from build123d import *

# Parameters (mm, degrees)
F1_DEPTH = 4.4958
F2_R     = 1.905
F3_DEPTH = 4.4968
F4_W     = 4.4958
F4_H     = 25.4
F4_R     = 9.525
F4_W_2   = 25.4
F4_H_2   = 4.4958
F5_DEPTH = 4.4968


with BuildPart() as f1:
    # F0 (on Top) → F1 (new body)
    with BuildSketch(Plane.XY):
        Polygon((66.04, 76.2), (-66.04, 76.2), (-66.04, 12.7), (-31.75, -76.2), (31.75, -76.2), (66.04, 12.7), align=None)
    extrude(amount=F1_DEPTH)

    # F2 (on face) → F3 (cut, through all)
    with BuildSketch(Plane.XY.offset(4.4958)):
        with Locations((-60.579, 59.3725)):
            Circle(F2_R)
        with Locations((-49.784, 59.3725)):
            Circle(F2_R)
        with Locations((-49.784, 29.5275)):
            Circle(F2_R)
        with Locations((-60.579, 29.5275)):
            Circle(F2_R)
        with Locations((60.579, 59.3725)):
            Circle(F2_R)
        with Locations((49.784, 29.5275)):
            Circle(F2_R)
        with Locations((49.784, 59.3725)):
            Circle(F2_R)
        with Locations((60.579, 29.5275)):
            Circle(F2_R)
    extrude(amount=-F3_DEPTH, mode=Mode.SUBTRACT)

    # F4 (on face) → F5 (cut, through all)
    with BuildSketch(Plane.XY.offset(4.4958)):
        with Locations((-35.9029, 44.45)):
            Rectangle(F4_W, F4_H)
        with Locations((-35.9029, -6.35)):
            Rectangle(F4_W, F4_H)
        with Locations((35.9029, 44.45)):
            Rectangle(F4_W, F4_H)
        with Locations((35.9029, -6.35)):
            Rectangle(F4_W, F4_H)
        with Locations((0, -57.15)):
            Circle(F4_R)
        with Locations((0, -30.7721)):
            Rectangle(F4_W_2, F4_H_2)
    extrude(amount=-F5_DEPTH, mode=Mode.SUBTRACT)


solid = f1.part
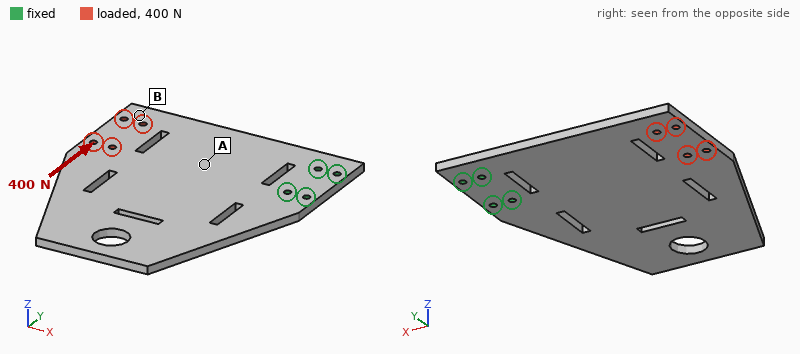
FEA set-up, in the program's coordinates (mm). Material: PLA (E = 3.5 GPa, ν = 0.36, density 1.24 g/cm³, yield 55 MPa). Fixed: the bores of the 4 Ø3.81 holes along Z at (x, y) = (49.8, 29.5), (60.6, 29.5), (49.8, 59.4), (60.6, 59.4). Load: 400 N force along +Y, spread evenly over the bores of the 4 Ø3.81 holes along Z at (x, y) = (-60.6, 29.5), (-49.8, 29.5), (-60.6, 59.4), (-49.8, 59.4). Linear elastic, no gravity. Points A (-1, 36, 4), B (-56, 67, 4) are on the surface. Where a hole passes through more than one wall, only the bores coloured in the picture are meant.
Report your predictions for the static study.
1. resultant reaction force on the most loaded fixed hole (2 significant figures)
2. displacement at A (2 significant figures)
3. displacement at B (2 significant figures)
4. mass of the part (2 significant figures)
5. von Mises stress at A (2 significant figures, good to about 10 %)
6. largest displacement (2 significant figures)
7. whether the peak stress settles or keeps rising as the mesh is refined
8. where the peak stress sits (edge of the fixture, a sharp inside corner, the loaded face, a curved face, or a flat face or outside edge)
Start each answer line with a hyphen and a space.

- 910 N
- 0.38 mm
- 0.84 mm
- 90 g
- 3.7 MPa
- 1.0 mm
- keeps rising
- edge of the fixture
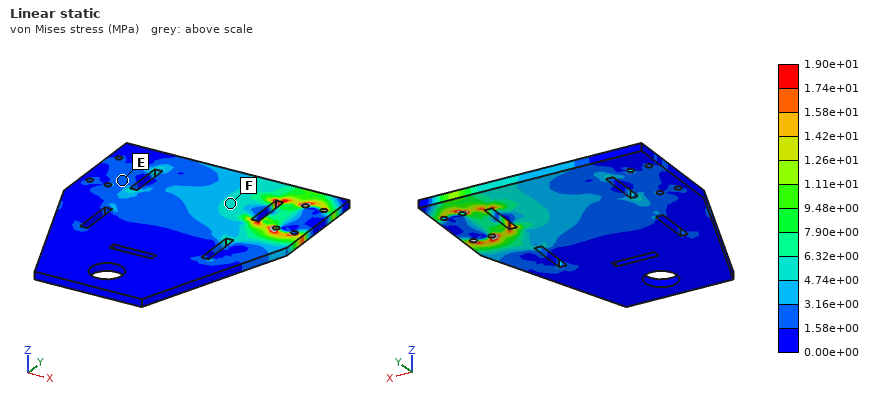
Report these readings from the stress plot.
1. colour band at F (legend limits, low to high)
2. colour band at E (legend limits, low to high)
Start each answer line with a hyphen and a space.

- 4.74e+00 to 6.32e+00 MPa
- 1.58e+00 to 3.16e+00 MPa
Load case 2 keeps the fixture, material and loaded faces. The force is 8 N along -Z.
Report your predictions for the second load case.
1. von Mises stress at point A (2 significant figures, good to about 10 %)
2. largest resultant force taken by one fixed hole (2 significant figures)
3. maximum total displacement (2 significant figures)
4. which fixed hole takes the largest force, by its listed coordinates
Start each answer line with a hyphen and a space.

- 1.1 MPa
- 29 N
- 1.9 mm
- (49.8, 29.5)
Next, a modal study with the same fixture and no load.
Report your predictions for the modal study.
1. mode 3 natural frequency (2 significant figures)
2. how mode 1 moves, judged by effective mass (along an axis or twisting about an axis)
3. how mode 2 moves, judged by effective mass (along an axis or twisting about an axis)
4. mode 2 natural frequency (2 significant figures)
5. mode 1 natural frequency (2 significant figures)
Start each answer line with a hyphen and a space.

- 300 Hz
- along Z
- twisting about X
- 110 Hz
- 66 Hz
